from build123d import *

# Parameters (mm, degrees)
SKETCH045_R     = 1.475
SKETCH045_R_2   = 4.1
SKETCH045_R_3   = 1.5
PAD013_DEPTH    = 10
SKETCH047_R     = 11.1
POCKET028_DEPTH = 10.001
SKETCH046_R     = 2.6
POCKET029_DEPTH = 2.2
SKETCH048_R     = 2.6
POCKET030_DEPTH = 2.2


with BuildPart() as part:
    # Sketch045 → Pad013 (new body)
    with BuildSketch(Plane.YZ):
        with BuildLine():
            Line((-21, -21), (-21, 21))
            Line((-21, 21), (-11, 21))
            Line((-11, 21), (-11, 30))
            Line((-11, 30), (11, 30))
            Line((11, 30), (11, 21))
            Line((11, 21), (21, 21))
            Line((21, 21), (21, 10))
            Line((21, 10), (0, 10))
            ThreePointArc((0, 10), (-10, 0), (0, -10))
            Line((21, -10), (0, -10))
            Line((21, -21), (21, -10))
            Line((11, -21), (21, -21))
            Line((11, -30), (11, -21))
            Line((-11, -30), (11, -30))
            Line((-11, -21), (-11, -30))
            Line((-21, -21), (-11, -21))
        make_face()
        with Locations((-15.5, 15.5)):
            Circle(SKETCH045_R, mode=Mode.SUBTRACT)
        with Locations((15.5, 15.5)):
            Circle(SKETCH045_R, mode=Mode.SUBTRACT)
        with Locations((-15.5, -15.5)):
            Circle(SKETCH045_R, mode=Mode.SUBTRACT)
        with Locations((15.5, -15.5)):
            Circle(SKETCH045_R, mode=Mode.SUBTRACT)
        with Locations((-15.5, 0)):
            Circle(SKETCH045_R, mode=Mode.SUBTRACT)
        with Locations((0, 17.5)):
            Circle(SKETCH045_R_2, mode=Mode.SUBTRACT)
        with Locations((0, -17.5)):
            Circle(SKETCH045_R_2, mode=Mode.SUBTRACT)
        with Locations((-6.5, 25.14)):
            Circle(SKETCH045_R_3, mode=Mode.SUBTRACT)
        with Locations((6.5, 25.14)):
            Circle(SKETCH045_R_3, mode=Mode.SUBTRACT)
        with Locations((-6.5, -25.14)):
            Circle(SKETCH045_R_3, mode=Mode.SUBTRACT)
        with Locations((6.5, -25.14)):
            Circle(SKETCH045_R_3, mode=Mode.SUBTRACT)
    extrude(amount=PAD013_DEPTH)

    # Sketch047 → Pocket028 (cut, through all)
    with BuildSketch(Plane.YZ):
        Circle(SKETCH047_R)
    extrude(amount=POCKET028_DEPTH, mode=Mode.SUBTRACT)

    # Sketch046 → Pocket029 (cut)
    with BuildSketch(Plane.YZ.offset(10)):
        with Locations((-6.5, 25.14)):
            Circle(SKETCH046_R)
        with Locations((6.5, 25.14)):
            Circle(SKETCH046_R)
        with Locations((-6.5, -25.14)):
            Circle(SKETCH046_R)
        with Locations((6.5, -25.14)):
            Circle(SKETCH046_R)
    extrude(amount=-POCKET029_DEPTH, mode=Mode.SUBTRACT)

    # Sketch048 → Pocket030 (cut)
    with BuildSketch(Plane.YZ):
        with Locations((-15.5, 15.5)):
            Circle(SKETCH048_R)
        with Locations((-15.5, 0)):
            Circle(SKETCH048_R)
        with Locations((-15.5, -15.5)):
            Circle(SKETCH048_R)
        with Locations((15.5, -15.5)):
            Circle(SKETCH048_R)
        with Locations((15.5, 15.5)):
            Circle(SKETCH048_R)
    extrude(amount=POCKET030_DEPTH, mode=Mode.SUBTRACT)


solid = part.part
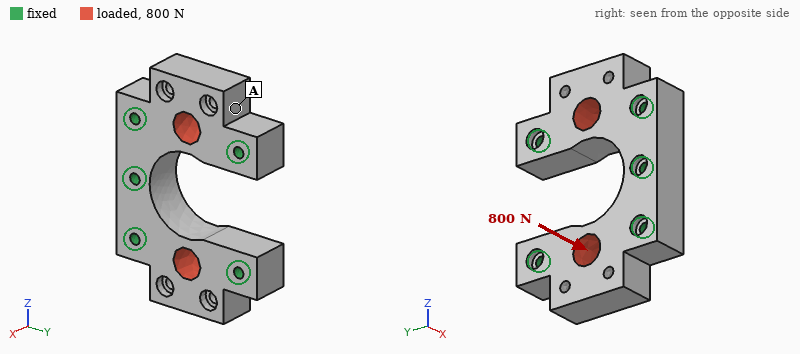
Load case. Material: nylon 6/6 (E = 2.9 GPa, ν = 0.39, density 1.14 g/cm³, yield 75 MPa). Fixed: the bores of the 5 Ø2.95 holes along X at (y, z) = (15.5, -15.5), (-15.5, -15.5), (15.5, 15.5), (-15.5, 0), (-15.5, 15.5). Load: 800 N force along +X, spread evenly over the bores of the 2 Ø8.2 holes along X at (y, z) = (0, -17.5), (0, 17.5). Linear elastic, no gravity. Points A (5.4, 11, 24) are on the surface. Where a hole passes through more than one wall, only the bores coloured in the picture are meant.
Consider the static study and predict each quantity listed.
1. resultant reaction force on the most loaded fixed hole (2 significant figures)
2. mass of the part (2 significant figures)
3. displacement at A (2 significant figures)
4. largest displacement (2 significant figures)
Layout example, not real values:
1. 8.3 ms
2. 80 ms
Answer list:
1. 210 N
2. 15 g
3. 42 µm
4. 74 µm
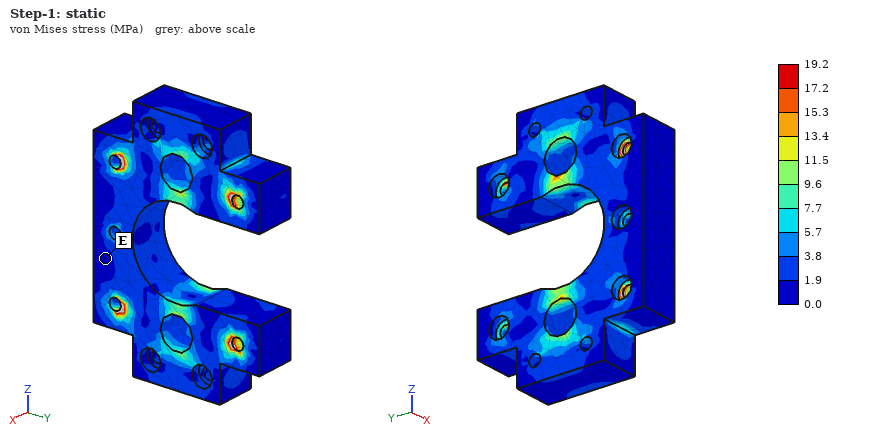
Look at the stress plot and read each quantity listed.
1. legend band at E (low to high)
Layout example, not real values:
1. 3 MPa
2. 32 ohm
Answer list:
1. 0.0 to 1.9 MPa
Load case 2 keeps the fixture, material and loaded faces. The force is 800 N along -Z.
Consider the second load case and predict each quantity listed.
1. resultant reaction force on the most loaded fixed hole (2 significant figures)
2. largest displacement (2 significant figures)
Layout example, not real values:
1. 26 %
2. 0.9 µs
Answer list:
1. 180 N
2. 44 µm
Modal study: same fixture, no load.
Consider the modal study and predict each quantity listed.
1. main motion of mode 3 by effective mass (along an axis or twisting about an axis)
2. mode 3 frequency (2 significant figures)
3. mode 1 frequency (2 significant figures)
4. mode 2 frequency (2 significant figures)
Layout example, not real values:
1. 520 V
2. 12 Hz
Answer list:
1. along Z
2. 10 kHz
3. 5300 Hz
4. 5300 Hz
